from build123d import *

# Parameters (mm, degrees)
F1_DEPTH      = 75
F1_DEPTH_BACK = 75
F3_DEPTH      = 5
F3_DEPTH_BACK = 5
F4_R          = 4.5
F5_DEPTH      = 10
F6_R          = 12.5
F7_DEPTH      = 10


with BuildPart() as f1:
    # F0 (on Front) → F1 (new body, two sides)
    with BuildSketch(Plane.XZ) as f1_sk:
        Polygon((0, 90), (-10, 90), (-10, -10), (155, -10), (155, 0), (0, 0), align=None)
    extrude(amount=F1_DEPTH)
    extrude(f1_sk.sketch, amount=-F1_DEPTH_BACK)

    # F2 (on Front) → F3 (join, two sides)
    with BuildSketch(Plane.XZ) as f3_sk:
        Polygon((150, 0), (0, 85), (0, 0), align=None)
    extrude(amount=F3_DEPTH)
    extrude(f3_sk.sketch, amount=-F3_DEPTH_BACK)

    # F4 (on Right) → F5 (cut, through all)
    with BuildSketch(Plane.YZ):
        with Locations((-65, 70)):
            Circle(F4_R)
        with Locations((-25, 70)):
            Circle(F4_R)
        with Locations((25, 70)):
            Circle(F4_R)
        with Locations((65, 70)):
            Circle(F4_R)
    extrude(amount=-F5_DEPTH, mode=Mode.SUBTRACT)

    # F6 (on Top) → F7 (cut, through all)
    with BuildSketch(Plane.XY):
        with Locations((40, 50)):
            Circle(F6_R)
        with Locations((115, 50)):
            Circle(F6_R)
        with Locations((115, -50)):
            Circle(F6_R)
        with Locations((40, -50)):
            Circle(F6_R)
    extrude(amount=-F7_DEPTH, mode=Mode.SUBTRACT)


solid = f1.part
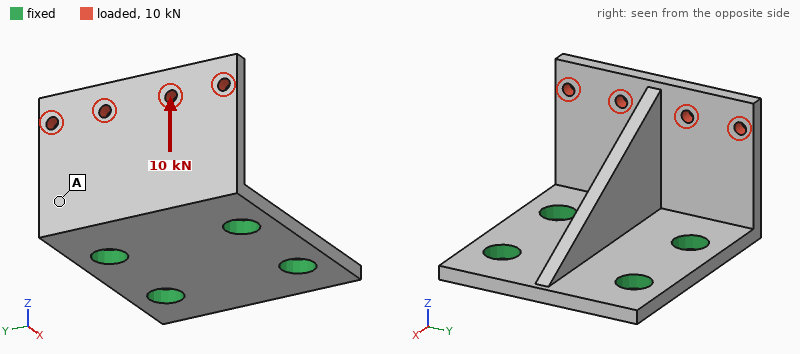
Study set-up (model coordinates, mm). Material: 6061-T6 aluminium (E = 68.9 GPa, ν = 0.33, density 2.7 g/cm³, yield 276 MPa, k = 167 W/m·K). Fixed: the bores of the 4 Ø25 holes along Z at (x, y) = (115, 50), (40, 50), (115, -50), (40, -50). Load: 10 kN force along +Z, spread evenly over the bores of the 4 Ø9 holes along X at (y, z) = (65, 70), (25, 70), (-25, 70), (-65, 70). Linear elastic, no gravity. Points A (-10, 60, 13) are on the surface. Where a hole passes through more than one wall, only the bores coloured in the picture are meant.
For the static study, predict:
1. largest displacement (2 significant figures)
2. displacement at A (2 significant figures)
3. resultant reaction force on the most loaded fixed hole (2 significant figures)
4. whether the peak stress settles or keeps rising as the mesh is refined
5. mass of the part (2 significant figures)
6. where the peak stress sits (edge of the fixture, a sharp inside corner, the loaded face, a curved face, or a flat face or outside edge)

0.21 mm
0.13 mm
6.3 kN
keeps rising
1.1 kg
edge of the fixture
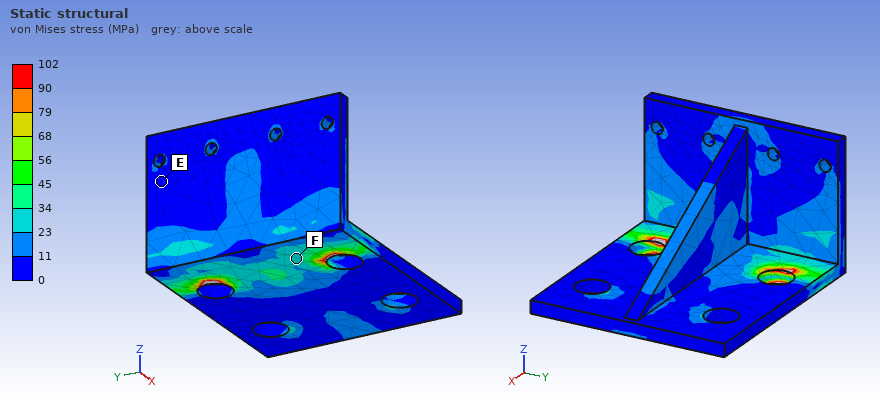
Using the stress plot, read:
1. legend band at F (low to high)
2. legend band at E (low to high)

23 to 34 MPa
0 to 11 MPa
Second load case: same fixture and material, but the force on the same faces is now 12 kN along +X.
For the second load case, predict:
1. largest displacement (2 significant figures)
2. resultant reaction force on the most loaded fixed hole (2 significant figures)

1.0 mm
5.5 kN
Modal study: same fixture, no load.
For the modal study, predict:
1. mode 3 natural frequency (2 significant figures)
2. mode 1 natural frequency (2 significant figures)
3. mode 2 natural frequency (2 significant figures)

2000 Hz
1400 Hz
1500 Hz
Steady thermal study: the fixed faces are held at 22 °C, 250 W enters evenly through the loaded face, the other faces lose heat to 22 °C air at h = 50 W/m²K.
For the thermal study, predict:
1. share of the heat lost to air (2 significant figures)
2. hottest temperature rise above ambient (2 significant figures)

38 %
79 K
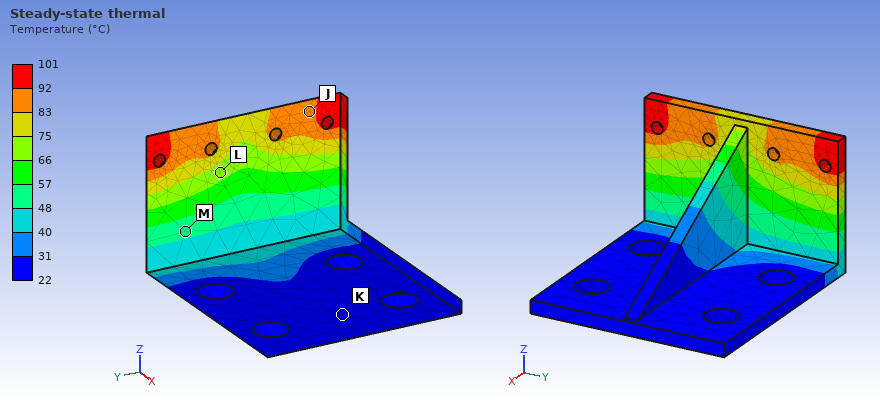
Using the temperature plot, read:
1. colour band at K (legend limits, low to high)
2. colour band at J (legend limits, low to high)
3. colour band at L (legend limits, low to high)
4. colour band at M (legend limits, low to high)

22 to 31 °C
83 to 92 °C
66 to 75 °C
48 to 57 °C
